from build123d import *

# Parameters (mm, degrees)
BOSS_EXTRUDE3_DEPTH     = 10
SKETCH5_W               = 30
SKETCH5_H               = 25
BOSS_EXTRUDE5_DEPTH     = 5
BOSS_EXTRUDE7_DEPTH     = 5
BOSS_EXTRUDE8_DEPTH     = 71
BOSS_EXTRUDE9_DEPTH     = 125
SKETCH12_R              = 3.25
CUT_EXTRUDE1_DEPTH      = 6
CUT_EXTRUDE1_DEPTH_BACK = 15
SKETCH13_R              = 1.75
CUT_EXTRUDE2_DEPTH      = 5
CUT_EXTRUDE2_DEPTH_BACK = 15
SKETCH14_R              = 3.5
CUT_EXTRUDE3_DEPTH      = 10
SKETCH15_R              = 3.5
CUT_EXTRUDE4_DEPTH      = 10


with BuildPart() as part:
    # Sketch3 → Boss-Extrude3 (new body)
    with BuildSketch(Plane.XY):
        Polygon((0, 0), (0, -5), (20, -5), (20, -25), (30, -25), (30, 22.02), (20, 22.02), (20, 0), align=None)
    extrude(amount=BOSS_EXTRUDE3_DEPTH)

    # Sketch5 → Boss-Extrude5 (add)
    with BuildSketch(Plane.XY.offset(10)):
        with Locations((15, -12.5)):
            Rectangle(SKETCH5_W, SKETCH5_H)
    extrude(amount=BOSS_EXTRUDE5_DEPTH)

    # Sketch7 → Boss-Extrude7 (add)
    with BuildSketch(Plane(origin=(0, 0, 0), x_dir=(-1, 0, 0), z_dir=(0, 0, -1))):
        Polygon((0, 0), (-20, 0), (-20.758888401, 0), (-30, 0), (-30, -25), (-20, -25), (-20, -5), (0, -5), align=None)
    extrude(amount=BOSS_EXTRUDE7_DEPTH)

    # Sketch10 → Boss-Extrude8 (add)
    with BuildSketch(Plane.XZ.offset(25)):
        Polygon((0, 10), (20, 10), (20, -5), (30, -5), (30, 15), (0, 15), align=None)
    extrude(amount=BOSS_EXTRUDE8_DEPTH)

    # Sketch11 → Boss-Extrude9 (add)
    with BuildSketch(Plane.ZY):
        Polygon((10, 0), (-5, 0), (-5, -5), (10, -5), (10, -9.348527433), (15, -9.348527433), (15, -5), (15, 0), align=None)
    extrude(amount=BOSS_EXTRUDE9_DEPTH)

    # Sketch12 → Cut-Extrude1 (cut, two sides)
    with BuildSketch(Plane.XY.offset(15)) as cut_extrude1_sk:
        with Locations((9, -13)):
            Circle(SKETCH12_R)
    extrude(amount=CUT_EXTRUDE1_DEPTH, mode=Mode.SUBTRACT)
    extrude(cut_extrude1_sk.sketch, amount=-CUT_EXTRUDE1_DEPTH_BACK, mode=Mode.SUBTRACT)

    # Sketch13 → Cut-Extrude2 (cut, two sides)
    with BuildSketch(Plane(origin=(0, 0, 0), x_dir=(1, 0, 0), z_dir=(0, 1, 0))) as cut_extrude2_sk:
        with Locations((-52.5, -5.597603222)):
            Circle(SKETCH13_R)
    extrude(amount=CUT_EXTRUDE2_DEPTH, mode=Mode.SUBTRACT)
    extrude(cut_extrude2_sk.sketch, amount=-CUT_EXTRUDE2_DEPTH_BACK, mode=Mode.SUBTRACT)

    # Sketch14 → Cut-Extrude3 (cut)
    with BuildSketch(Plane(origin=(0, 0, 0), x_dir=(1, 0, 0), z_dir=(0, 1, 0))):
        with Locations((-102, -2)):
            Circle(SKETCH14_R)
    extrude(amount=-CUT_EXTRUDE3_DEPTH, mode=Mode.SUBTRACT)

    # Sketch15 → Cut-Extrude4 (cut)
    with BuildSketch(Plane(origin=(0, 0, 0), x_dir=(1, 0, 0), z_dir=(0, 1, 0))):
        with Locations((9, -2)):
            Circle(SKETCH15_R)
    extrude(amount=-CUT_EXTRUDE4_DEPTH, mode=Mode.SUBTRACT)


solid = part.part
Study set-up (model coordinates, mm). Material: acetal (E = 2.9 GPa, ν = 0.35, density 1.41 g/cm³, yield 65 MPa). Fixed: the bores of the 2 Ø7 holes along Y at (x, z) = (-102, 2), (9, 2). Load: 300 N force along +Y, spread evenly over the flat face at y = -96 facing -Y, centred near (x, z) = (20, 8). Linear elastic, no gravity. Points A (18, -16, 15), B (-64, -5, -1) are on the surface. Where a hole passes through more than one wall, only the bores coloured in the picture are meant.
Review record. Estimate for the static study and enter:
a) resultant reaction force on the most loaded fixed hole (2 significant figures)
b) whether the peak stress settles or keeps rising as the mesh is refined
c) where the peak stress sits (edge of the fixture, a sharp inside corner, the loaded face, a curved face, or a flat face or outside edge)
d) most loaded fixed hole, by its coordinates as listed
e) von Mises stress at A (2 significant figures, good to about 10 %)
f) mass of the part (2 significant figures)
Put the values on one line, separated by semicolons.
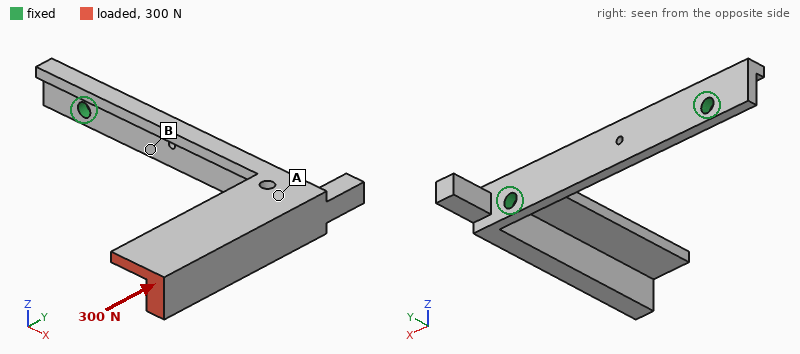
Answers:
310 N; keeps rising; edge of the fixture; (9, 2); 2.7 MPa; 66 g
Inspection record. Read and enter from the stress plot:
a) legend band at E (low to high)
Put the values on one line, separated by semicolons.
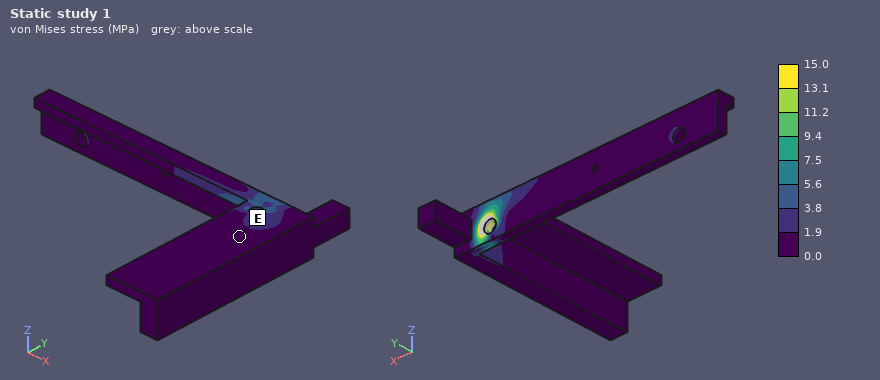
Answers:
0.0 to 1.9 MPa
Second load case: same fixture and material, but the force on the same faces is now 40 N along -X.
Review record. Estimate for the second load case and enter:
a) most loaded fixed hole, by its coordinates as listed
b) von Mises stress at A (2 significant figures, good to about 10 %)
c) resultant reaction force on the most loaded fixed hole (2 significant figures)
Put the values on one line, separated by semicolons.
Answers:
(-102, 2); 2.9 MPa; 38 N
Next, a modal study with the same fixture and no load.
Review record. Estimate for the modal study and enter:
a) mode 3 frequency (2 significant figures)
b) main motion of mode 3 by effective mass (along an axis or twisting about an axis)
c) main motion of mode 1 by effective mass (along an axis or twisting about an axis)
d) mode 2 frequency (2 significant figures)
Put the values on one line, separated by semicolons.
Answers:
830 Hz; along Y; along Z; 240 Hz
